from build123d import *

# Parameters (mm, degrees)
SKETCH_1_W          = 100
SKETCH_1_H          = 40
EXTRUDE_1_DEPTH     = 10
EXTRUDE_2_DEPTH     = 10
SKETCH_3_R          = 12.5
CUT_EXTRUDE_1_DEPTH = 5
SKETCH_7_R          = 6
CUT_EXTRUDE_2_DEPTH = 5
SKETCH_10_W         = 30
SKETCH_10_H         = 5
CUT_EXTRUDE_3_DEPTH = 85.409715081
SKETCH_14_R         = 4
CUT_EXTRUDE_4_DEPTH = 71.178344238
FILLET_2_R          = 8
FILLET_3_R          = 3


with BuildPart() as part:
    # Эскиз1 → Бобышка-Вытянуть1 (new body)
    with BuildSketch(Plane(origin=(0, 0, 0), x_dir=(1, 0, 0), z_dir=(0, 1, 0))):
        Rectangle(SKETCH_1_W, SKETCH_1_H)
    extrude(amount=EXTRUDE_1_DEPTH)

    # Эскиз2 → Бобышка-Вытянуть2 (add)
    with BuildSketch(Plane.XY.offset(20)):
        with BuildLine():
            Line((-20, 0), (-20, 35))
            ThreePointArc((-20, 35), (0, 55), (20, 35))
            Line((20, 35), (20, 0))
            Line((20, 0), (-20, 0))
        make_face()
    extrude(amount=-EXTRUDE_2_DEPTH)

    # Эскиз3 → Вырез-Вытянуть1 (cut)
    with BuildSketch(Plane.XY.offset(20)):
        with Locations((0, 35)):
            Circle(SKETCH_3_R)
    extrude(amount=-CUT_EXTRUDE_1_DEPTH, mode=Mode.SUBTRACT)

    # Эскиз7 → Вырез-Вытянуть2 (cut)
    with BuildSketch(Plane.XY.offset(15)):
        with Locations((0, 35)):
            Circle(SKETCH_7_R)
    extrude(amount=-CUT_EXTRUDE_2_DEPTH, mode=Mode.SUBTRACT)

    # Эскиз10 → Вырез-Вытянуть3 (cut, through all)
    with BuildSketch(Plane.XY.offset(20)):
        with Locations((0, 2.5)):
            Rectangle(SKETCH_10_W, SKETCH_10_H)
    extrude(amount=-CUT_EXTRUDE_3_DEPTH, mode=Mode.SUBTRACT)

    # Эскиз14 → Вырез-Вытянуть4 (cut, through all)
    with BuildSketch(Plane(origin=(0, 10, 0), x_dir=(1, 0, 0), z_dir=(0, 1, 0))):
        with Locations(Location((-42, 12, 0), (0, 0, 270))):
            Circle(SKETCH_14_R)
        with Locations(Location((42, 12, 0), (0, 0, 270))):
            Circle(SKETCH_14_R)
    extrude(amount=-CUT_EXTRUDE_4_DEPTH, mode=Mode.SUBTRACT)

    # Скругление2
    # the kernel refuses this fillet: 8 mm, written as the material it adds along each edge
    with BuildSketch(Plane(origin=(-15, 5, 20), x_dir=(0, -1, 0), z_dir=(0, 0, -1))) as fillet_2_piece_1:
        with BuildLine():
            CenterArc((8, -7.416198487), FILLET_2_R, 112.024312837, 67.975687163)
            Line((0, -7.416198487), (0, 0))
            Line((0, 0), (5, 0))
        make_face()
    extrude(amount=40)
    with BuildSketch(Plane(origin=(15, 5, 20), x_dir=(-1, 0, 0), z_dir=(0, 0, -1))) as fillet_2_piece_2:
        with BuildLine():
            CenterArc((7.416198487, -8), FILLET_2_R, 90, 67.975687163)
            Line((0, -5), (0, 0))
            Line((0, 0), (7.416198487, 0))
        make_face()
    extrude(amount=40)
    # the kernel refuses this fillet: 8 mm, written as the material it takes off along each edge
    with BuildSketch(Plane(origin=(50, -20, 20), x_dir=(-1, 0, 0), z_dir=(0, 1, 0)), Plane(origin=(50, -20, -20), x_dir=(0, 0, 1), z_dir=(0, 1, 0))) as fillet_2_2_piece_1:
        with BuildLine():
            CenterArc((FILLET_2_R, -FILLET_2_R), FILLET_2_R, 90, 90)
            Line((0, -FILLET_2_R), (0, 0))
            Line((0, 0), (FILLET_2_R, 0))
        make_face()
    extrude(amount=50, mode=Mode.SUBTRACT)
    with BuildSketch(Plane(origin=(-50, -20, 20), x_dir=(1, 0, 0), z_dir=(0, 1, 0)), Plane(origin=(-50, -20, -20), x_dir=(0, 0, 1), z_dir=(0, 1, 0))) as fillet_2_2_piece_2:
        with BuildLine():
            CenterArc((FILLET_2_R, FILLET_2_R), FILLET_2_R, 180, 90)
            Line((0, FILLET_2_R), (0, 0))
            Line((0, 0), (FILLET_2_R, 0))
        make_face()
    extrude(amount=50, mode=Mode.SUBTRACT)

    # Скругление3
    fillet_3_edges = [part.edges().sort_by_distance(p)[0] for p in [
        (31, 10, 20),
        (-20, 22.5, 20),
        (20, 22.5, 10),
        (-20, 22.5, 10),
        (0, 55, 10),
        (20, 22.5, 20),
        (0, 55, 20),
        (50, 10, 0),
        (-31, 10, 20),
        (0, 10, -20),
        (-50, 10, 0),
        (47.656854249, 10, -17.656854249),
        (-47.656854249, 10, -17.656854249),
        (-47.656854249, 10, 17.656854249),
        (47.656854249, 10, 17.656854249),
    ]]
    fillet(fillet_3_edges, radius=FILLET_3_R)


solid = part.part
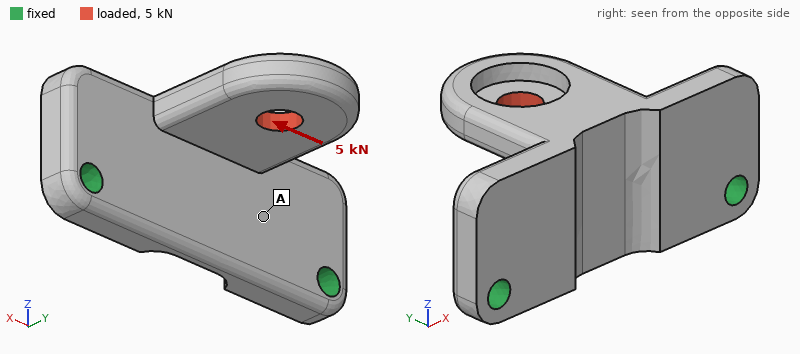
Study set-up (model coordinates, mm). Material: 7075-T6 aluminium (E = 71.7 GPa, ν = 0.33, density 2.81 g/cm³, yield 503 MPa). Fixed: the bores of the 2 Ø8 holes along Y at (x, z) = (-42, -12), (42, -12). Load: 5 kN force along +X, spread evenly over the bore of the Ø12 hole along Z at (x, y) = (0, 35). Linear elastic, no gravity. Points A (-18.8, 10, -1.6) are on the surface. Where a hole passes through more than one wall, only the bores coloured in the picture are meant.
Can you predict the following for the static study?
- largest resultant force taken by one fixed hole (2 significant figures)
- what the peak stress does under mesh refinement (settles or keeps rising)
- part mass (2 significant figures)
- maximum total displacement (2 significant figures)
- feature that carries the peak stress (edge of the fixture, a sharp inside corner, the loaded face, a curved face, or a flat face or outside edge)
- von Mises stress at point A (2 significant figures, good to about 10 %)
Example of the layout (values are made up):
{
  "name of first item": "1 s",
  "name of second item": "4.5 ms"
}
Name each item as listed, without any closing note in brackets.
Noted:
{
  "largest resultant force taken by one fixed hole": "3.6 kN",
  "what the peak stress does under mesh refinement": "keeps rising",
  "part mass": "130 g",
  "maximum total displacement": "0.26 mm",
  "feature that carries the peak stress": "a sharp inside corner",
  "von Mises stress at point A": "47 MPa"
}
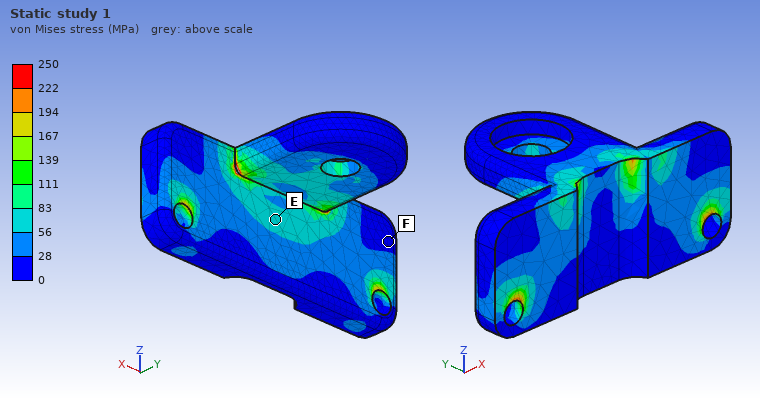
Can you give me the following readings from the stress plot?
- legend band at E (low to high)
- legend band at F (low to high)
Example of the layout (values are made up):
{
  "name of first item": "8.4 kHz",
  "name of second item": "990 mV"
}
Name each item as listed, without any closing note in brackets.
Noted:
{
  "legend band at E": "56 to 83 MPa",
  "legend band at F": "0 to 28 MPa"
}
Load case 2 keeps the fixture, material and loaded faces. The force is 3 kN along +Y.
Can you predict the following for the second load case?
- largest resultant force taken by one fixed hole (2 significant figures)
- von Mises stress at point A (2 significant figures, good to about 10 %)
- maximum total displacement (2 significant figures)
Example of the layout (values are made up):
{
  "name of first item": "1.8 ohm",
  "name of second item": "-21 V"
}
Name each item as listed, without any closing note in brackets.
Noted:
{
  "largest resultant force taken by one fixed hole": "1.7 kN",
  "von Mises stress at point A": "25 MPa",
  "maximum total displacement": "0.18 mm"
}
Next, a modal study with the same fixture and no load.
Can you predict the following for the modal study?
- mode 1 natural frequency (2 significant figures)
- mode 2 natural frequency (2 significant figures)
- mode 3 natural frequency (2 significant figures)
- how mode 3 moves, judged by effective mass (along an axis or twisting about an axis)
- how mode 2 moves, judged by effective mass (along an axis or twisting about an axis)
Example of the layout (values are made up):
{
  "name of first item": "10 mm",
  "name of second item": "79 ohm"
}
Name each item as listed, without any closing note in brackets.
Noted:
{
  "mode 1 natural frequency": "2200 Hz",
  "mode 2 natural frequency": "4200 Hz",
  "mode 3 natural frequency": "4400 Hz",
  "how mode 3 moves, judged by effective mass": "along X",
  "how mode 2 moves, judged by effective mass": "along Y"
}
